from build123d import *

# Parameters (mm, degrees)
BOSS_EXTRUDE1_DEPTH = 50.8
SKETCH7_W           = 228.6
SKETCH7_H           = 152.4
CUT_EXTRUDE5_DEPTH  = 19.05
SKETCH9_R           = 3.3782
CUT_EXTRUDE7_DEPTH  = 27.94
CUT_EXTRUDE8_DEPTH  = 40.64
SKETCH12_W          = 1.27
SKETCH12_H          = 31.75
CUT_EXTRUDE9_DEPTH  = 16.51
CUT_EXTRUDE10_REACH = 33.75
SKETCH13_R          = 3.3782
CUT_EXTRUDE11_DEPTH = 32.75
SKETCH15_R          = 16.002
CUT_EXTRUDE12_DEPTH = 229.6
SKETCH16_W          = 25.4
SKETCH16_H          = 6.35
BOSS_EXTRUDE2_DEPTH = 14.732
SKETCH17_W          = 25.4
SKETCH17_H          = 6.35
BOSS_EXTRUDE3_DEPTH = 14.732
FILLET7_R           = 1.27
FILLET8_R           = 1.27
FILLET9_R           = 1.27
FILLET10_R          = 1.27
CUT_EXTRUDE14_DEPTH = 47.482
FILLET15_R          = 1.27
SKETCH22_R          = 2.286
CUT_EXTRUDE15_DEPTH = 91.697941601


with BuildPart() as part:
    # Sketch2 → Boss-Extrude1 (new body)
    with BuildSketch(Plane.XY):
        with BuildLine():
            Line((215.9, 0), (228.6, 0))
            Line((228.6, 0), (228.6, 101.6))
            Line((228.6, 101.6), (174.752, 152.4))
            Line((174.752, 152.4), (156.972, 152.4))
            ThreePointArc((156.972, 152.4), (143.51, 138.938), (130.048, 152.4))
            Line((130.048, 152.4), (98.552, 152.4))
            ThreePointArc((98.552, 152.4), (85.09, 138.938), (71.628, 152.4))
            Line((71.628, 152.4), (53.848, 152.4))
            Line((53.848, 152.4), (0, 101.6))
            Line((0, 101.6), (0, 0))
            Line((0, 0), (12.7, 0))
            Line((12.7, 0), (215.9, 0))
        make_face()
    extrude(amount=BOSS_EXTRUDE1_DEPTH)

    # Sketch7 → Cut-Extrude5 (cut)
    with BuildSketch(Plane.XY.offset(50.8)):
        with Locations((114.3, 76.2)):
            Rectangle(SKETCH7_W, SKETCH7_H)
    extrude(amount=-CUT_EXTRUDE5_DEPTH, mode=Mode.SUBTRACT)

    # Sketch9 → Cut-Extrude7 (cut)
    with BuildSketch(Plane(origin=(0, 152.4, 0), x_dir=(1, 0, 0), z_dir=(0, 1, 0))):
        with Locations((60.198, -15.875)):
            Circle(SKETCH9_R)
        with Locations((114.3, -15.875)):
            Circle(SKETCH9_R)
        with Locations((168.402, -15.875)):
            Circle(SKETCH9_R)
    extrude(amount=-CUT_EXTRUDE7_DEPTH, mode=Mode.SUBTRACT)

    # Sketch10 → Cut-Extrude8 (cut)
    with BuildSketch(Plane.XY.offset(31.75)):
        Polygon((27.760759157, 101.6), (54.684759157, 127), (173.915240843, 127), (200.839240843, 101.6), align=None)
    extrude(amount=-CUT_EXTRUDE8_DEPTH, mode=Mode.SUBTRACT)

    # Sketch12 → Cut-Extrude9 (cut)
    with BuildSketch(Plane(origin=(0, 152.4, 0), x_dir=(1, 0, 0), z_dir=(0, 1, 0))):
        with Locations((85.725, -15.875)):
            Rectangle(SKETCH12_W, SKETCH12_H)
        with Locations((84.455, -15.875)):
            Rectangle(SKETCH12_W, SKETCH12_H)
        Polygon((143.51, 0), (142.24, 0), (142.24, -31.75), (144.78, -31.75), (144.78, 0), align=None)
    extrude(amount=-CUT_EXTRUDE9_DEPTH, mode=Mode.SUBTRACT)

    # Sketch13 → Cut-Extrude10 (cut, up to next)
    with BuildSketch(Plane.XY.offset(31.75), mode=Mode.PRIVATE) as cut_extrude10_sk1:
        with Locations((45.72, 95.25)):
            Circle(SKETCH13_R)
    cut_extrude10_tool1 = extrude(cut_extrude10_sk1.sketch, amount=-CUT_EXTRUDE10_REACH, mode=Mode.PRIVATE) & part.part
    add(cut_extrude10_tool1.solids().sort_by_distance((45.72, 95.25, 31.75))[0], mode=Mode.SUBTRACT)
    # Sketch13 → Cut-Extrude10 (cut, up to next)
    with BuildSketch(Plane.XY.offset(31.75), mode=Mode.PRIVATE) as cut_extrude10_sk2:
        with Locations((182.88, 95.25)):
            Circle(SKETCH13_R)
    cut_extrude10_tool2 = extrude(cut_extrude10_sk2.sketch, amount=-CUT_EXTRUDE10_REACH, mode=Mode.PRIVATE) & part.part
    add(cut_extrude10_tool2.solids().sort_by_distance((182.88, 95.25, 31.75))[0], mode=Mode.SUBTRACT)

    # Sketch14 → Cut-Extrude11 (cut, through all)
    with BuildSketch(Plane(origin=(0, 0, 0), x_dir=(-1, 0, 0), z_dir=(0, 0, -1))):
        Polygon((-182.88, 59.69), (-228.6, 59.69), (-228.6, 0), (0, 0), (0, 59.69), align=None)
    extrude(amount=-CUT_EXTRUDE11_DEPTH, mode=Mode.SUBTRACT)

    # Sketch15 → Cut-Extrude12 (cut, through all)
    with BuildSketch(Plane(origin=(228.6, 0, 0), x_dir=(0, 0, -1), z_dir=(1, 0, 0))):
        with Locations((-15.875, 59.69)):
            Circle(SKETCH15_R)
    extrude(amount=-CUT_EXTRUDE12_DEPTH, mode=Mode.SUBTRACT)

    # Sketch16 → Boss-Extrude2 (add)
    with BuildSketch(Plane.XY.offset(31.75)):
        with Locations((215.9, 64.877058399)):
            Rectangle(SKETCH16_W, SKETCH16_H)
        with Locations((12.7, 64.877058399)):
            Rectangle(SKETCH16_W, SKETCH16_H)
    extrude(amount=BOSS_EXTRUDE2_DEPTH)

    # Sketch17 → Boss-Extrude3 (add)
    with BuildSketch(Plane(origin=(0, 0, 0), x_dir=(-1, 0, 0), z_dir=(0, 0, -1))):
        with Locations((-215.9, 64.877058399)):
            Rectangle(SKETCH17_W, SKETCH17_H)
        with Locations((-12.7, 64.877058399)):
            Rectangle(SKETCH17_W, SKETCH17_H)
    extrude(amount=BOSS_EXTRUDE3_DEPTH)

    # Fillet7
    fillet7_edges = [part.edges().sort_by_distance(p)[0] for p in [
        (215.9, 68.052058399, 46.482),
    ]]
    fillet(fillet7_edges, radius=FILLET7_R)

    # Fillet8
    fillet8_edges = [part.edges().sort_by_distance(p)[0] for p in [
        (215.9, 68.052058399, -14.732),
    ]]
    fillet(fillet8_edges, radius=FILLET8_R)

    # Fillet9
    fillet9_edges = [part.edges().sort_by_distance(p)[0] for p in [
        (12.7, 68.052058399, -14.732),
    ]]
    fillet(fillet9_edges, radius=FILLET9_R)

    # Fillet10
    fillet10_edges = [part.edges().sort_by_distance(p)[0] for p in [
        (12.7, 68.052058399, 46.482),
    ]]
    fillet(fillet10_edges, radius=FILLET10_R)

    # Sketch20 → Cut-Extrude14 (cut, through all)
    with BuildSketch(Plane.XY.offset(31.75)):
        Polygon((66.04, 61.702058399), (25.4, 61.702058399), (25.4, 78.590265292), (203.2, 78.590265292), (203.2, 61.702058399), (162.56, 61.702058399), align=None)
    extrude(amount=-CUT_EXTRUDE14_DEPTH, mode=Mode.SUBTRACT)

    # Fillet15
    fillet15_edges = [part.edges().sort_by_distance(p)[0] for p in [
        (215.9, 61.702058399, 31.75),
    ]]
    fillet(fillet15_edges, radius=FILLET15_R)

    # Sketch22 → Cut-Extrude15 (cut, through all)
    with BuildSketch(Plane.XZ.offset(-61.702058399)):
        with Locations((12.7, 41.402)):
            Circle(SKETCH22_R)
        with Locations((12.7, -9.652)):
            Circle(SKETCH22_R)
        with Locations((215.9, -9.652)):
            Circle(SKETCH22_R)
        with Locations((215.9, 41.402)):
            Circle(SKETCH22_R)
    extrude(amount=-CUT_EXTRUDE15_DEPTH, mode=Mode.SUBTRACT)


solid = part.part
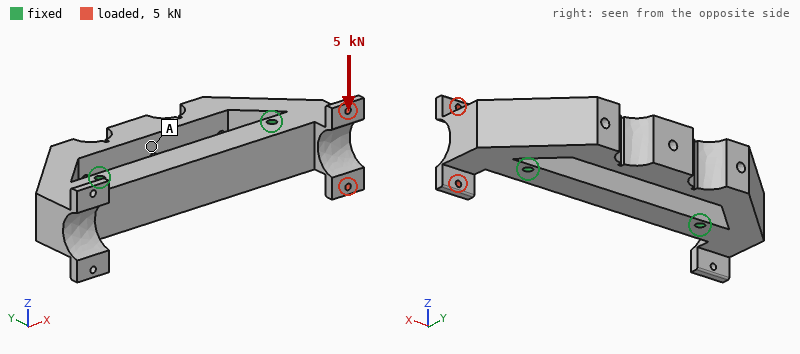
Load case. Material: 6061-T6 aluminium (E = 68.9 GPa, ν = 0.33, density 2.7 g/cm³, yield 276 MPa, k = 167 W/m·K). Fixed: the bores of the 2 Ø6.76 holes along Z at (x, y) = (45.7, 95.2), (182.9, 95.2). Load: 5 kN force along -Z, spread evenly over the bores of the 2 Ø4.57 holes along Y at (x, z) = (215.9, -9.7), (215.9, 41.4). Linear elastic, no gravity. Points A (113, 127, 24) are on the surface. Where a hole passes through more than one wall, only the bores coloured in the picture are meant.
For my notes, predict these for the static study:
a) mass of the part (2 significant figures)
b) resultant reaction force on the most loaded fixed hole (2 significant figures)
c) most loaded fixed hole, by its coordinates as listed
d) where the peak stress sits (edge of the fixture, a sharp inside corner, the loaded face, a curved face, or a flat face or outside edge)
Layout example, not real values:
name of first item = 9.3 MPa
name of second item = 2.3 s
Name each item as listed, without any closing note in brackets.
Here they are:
mass of the part = 880 g
resultant reaction force on the most loaded fixed hole = 5.3 kN
most loaded fixed hole, by its coordinates as listed = (182.9, 95.2)
where the peak stress sits = a curved face
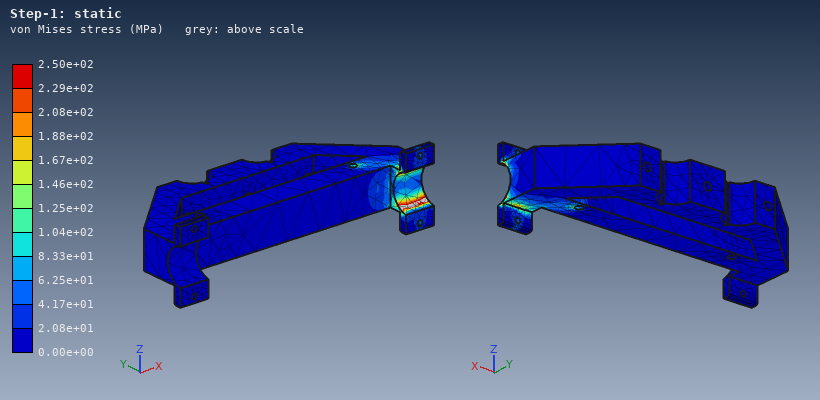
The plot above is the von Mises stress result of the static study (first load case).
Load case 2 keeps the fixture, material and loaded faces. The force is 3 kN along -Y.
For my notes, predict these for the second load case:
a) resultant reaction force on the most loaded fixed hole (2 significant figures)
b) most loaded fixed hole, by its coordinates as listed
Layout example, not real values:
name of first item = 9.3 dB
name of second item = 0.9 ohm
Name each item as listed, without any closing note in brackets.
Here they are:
resultant reaction force on the most loaded fixed hole = 3.3 kN
most loaded fixed hole, by its coordinates as listed = (182.9, 95.2)
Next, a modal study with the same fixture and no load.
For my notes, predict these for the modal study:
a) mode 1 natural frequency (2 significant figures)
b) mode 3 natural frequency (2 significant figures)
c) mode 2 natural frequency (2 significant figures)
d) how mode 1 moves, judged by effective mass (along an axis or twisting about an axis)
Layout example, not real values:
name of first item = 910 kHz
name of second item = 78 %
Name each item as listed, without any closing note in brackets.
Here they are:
mode 1 natural frequency = 1700 Hz
mode 3 natural frequency = 2400 Hz
mode 2 natural frequency = 2400 Hz
how mode 1 moves, judged by effective mass = along Z
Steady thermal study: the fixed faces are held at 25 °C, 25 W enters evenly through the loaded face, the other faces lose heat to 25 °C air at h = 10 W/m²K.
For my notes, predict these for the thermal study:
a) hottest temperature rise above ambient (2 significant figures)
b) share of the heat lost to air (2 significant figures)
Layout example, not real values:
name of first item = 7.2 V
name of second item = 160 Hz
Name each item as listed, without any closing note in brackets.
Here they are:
hottest temperature rise above ambient = 23 K
share of the heat lost to air = 5.2 %
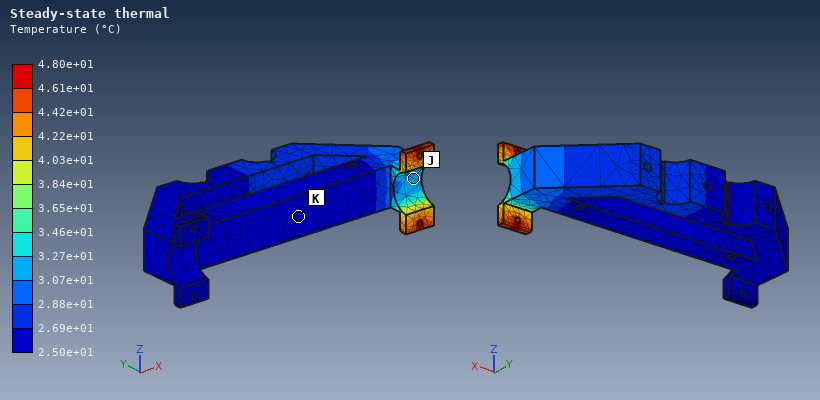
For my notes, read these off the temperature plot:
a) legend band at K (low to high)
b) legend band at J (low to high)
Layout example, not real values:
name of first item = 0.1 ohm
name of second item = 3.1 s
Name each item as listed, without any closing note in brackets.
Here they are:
legend band at K = 2.50e+01 to 2.69e+01 °C
legend band at J = 3.07e+01 to 3.27e+01 °C
